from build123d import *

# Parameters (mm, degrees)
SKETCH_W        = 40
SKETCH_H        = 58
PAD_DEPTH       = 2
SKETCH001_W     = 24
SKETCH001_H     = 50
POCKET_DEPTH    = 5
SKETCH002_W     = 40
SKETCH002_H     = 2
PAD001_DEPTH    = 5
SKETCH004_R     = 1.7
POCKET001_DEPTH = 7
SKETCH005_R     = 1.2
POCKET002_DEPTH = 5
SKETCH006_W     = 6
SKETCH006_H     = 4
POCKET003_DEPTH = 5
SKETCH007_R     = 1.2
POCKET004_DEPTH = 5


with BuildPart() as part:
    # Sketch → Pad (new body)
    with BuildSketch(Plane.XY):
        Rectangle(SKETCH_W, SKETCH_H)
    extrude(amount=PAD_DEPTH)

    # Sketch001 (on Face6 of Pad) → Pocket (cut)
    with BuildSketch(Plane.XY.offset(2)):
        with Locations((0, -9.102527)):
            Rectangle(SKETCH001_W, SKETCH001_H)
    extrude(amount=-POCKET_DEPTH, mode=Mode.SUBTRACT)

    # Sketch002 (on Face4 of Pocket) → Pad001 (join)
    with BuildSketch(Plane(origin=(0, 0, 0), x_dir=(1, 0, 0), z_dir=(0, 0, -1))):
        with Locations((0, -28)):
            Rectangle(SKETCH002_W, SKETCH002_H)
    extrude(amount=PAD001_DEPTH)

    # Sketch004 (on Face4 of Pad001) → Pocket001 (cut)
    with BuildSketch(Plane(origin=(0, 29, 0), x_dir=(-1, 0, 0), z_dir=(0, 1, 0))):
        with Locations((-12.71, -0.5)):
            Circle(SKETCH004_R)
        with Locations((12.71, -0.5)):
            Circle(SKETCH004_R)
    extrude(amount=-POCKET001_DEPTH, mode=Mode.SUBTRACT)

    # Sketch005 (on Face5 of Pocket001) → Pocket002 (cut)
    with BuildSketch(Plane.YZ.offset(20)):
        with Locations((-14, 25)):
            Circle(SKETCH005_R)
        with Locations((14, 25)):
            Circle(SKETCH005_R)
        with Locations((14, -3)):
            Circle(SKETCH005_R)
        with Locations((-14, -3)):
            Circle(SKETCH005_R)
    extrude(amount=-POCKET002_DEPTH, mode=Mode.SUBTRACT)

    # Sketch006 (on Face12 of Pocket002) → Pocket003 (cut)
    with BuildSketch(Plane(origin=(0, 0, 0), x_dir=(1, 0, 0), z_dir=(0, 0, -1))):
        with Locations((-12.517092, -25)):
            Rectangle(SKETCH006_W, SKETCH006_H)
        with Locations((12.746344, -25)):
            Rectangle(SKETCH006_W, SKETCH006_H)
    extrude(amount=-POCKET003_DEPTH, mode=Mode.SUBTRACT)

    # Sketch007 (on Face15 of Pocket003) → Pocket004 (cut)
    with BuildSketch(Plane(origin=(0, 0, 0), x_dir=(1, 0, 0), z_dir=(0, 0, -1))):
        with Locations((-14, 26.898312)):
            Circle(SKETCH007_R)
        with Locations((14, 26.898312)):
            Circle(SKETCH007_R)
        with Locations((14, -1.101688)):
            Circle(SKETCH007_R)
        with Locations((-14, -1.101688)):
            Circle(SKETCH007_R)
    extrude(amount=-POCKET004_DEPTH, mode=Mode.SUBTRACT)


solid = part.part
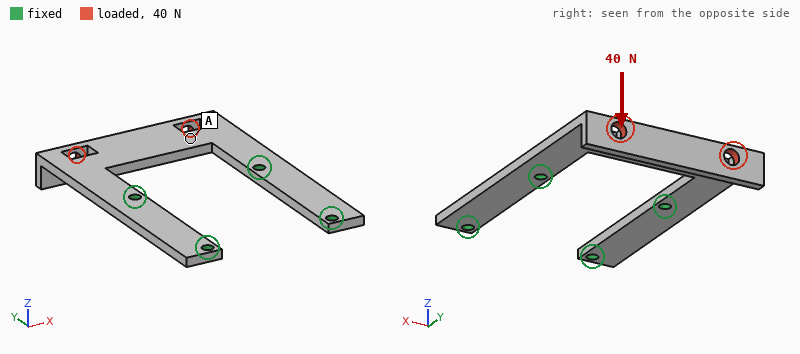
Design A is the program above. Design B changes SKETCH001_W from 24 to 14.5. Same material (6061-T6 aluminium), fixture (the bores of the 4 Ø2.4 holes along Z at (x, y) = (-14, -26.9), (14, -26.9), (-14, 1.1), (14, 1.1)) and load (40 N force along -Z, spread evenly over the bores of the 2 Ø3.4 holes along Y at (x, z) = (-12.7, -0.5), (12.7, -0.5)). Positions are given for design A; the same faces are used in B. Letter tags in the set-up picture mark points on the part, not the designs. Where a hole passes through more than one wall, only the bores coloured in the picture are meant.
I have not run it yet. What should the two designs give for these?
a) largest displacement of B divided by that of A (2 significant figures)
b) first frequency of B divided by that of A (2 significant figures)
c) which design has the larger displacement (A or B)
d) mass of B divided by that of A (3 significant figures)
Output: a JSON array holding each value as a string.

["0.64", "1.2", "A", "1.31"]
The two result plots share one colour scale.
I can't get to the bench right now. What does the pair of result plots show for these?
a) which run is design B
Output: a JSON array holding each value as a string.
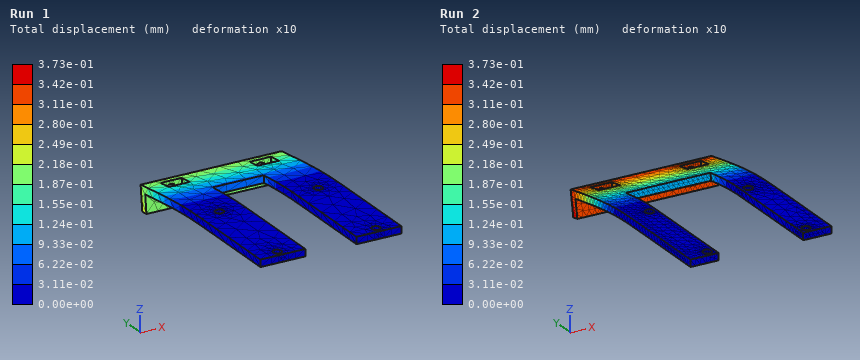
["Run 1"]
